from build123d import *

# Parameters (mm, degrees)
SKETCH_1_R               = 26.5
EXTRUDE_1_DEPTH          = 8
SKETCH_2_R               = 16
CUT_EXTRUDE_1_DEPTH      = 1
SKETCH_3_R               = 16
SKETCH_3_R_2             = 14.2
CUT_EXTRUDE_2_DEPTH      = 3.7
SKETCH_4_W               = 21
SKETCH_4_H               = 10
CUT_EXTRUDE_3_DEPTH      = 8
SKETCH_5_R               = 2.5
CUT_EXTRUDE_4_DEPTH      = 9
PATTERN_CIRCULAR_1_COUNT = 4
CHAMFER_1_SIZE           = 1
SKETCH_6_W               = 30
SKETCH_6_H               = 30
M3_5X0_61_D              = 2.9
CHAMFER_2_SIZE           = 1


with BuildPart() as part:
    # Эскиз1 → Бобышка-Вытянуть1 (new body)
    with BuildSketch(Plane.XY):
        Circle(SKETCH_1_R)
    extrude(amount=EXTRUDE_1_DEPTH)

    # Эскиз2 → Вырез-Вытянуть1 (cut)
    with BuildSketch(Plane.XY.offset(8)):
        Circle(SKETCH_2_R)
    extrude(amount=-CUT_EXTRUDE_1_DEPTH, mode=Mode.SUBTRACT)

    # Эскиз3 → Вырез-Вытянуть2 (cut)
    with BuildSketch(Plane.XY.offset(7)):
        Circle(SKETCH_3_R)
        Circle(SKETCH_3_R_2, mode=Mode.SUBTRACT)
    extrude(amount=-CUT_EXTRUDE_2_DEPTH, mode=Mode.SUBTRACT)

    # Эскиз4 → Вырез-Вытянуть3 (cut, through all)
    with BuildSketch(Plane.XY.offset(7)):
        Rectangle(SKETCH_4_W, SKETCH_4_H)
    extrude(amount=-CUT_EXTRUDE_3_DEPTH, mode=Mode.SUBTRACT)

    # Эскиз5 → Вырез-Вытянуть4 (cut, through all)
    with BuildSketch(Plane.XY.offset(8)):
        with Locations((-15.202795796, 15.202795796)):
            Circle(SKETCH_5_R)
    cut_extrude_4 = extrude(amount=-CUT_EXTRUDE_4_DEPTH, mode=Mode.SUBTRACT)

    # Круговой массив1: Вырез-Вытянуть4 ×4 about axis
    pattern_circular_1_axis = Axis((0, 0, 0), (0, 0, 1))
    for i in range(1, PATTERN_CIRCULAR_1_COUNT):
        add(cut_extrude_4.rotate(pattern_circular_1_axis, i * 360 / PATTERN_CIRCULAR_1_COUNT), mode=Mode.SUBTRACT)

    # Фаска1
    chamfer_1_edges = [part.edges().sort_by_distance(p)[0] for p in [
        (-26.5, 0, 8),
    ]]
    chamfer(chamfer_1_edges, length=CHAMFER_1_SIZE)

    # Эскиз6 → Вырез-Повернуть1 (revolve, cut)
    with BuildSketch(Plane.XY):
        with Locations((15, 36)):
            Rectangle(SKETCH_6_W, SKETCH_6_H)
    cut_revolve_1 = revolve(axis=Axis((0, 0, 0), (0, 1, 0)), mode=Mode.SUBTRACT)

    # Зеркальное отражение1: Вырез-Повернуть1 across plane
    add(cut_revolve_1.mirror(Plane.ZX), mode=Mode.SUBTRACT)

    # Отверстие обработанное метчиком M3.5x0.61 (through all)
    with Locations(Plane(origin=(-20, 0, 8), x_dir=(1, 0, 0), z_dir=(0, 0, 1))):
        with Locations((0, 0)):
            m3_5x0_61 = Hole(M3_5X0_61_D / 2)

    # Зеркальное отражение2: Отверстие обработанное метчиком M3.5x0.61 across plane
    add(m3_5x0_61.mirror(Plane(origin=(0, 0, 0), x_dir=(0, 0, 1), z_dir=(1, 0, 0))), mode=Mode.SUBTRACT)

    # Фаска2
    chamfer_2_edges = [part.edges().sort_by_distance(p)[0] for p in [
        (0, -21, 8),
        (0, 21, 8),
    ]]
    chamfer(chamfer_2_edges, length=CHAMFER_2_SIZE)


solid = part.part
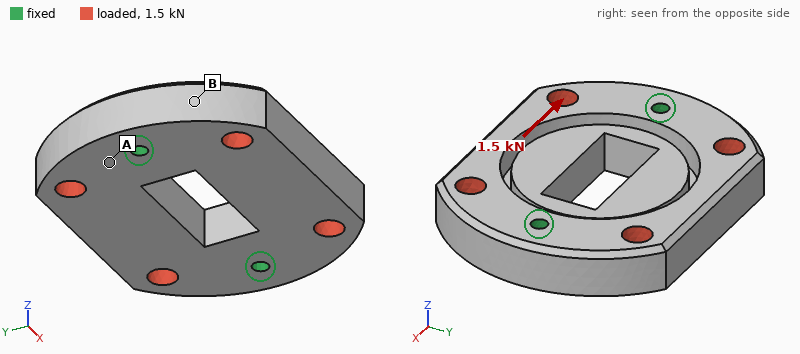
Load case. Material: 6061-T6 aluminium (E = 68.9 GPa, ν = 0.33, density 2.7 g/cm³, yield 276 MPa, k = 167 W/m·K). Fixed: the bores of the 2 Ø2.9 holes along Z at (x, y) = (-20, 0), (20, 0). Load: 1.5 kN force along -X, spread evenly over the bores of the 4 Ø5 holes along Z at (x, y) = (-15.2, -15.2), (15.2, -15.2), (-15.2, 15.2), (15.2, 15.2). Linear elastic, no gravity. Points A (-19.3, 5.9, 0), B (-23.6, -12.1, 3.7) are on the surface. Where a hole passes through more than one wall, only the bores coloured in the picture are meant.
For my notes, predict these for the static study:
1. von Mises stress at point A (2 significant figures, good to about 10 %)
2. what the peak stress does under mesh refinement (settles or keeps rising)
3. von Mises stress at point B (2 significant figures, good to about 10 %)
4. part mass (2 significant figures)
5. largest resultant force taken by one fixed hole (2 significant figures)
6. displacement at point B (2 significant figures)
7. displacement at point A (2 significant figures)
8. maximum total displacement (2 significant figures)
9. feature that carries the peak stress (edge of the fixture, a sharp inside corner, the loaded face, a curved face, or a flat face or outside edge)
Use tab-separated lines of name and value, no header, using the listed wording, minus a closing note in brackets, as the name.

von Mises stress at point A	5.5 MPa
what the peak stress does under mesh refinement	keeps rising
von Mises stress at point B	2.7 MPa
part mass	32 g
largest resultant force taken by one fixed hole	750 N
displacement at point B	2.7 µm
displacement at point A	1.2 µm
maximum total displacement	4.0 µm
feature that carries the peak stress	edge of the fixture
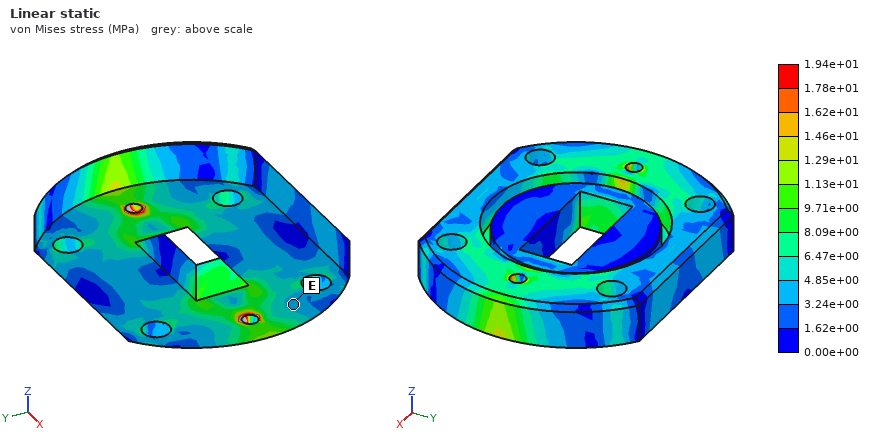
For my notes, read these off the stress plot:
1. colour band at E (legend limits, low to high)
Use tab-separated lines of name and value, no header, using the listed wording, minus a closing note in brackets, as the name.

colour band at E	3.24e+00 to 4.85e+00 MPa
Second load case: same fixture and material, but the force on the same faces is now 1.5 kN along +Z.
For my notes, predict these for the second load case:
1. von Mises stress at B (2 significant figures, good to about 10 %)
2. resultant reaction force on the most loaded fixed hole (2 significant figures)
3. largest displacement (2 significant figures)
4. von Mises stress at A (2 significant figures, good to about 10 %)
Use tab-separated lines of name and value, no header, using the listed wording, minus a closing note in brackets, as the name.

von Mises stress at B	9.8 MPa
resultant reaction force on the most loaded fixed hole	760 N
largest displacement	24 µm
von Mises stress at A	24 MPa
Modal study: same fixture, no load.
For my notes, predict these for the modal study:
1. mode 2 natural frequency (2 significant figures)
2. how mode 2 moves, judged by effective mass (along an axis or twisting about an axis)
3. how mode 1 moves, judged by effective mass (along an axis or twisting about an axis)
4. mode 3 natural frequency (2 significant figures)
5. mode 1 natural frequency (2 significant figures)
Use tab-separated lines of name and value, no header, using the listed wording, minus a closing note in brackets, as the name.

mode 2 natural frequency	9900 Hz
how mode 2 moves, judged by effective mass	along Z
how mode 1 moves, judged by effective mass	twisting about X
mode 3 natural frequency	17 kHz
mode 1 natural frequency	8500 Hz
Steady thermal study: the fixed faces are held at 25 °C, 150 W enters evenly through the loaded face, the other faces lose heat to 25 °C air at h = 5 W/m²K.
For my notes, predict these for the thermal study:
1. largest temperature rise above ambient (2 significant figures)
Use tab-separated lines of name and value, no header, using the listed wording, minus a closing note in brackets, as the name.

largest temperature rise above ambient	44 K
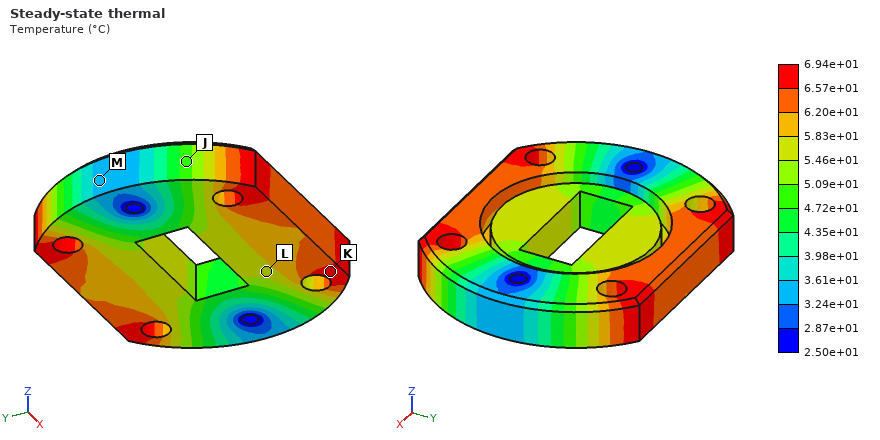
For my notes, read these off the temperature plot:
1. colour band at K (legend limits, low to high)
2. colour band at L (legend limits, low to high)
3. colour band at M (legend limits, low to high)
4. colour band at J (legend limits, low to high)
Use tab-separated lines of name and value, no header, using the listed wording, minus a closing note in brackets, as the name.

colour band at K	6.57e+01 to 6.94e+01 °C
colour band at L	5.46e+01 to 5.83e+01 °C
colour band at M	3.24e+01 to 3.61e+01 °C
colour band at J	4.72e+01 to 5.09e+01 °C
